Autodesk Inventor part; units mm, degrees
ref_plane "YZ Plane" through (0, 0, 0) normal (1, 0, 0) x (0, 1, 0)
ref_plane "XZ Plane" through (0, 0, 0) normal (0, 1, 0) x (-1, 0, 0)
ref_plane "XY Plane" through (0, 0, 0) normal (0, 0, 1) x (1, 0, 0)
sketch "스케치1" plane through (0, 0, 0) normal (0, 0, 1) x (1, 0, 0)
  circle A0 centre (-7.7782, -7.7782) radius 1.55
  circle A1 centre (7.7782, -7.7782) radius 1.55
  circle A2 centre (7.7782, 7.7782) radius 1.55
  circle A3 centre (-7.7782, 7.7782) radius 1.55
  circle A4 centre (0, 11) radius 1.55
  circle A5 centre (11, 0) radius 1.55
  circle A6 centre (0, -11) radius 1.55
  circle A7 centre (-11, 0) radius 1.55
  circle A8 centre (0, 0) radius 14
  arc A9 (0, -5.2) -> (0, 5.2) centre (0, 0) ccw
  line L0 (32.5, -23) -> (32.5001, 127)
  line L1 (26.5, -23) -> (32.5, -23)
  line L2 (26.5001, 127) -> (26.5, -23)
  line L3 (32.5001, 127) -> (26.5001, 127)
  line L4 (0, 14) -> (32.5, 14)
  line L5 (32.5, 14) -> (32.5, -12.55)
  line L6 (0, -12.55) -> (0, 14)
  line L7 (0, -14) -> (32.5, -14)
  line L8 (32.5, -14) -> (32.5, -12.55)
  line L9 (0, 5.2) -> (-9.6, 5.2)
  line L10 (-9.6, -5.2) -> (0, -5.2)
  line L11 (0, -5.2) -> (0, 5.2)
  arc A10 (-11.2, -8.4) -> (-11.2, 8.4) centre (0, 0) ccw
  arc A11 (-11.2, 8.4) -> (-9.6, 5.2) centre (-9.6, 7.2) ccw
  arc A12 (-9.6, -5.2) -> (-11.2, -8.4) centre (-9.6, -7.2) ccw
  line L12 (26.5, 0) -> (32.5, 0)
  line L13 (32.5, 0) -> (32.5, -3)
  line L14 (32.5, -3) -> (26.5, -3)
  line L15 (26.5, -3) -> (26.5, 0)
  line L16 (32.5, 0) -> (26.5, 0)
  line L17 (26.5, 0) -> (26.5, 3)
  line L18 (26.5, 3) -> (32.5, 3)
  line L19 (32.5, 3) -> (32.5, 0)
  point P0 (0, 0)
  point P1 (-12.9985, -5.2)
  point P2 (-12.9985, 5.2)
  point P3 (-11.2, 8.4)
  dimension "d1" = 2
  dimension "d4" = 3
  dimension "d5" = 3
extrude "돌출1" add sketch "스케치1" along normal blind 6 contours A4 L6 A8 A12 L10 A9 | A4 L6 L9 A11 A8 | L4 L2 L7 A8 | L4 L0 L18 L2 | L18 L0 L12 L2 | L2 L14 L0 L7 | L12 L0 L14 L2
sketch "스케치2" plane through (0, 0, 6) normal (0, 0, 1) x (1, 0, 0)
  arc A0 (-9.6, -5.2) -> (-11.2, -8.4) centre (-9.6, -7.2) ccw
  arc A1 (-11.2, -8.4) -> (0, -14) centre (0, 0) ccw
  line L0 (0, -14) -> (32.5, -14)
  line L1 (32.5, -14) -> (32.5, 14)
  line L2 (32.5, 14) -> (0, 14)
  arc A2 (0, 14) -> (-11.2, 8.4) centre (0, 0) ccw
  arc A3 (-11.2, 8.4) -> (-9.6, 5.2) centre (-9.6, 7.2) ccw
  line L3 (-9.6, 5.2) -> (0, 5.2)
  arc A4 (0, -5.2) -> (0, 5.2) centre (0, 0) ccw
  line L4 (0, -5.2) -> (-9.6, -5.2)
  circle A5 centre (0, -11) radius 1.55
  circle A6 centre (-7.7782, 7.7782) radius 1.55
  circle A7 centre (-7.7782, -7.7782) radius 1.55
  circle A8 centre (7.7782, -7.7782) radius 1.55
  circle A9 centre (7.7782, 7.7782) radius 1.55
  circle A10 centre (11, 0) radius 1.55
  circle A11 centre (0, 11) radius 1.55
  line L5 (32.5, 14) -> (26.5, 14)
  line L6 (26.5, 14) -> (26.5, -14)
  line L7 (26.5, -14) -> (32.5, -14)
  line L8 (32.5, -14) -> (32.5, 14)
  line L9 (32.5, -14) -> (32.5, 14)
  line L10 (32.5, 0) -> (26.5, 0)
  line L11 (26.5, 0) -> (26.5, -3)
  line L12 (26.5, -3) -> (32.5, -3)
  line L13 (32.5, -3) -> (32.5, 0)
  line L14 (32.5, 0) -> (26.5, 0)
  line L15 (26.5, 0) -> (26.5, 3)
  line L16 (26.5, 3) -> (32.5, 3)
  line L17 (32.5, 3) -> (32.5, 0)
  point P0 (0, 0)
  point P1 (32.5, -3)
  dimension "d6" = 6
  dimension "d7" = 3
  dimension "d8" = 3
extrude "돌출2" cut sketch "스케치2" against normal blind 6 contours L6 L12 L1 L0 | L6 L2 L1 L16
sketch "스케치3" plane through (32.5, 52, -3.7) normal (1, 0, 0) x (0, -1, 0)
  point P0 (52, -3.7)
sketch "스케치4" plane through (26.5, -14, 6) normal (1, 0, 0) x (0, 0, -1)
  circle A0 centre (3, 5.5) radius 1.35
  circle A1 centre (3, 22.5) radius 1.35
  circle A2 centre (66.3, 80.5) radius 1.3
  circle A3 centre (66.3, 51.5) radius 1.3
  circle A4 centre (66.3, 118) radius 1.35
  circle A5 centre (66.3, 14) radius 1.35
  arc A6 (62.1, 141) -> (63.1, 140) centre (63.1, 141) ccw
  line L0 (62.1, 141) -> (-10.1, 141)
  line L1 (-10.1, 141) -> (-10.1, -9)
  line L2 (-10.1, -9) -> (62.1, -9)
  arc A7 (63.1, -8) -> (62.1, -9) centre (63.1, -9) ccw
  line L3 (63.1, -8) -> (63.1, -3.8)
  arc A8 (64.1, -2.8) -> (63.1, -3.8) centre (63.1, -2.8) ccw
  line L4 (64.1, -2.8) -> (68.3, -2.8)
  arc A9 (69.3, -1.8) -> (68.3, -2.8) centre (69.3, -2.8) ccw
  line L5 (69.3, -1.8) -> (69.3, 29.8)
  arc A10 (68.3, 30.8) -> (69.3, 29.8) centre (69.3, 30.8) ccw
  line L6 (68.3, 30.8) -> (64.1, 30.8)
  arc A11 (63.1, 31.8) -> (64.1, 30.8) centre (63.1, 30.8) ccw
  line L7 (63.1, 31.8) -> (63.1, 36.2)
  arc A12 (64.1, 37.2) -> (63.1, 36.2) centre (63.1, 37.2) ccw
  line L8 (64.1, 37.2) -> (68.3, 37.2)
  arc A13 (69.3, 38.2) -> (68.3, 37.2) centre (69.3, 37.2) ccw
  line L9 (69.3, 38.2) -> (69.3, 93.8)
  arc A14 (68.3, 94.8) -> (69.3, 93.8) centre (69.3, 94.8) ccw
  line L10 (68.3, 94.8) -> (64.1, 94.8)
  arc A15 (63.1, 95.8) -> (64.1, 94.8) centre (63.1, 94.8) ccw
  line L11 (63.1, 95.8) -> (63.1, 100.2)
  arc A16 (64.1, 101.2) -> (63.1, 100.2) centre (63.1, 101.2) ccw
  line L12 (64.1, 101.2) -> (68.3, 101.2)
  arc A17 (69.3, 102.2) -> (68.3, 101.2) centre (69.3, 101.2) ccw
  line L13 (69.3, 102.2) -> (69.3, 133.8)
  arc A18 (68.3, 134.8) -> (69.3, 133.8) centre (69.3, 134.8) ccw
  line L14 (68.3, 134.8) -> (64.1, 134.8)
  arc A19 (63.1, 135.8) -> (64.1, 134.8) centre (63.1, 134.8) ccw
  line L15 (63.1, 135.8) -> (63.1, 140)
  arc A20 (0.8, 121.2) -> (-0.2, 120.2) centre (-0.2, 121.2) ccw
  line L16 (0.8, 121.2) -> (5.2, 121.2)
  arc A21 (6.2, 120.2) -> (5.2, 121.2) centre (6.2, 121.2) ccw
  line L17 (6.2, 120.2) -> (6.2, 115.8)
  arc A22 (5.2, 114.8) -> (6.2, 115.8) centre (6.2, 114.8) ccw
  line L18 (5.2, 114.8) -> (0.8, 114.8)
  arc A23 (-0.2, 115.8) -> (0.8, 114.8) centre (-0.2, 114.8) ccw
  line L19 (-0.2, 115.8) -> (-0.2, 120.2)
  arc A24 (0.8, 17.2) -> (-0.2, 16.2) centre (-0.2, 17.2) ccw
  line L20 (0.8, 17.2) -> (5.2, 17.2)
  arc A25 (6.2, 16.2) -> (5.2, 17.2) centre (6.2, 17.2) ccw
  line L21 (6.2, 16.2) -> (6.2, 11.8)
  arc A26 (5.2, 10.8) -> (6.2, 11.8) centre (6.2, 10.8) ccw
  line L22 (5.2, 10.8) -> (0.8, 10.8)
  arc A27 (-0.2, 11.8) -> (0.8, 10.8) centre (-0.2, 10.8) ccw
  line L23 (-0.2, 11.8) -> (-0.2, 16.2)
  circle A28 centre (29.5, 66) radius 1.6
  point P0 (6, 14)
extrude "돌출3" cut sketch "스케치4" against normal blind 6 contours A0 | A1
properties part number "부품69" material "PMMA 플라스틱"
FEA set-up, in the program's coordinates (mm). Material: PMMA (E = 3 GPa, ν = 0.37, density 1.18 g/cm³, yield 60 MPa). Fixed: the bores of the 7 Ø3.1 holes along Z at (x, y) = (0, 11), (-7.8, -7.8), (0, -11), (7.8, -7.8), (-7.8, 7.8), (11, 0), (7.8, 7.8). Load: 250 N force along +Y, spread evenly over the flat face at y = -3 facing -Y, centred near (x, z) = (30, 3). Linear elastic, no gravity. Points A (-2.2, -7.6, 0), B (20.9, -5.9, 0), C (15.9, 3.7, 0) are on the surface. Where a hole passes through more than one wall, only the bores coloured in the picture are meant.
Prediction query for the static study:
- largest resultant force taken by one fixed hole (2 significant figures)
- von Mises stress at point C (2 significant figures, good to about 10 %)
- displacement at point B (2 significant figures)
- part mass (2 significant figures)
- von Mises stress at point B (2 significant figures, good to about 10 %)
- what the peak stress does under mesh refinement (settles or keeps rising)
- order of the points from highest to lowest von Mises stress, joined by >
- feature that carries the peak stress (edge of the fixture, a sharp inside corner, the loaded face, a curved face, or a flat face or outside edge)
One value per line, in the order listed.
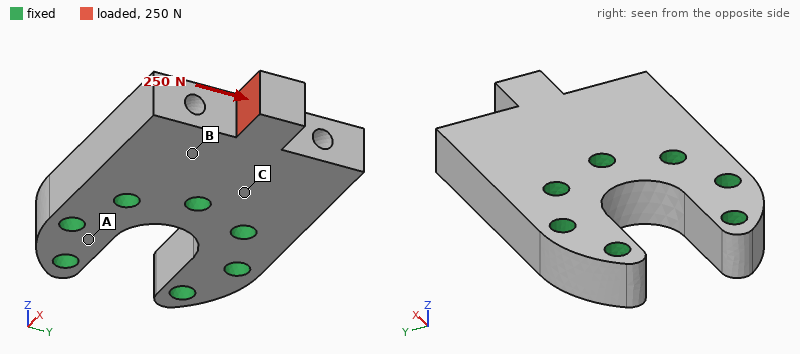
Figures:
190 N
4.3 MPa
0.033 mm
5.9 g
5.7 MPa
keeps rising
B > C > A
a sharp inside corner
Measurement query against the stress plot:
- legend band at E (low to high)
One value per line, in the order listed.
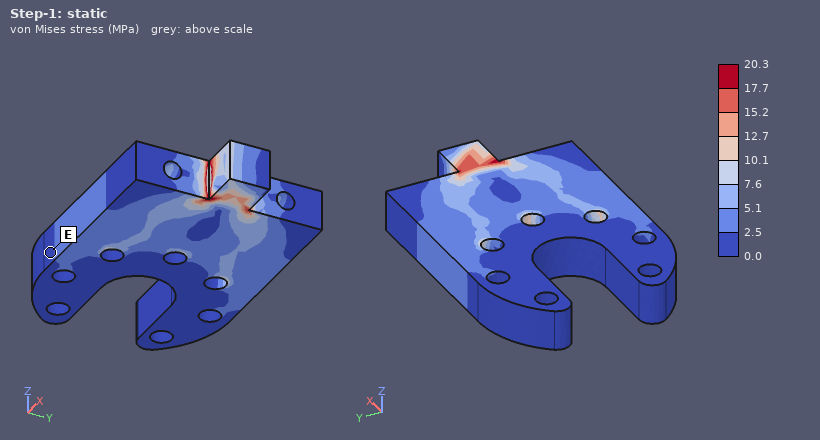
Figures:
0.0 to 2.5 MPa
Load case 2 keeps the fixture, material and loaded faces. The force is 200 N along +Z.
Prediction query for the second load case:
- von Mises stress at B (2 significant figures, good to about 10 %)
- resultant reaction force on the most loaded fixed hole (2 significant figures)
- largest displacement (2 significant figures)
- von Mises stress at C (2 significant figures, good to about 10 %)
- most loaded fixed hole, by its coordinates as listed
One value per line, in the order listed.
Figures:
13 MPa
250 N
0.63 mm
17 MPa
(11, 0)
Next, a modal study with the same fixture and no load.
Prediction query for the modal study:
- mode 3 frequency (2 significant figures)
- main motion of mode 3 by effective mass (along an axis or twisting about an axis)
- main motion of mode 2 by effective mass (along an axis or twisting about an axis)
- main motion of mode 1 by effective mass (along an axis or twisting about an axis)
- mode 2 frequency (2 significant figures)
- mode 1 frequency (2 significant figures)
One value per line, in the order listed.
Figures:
9300 Hz
along Y
twisting about X
along Z
7000 Hz
4300 Hz
